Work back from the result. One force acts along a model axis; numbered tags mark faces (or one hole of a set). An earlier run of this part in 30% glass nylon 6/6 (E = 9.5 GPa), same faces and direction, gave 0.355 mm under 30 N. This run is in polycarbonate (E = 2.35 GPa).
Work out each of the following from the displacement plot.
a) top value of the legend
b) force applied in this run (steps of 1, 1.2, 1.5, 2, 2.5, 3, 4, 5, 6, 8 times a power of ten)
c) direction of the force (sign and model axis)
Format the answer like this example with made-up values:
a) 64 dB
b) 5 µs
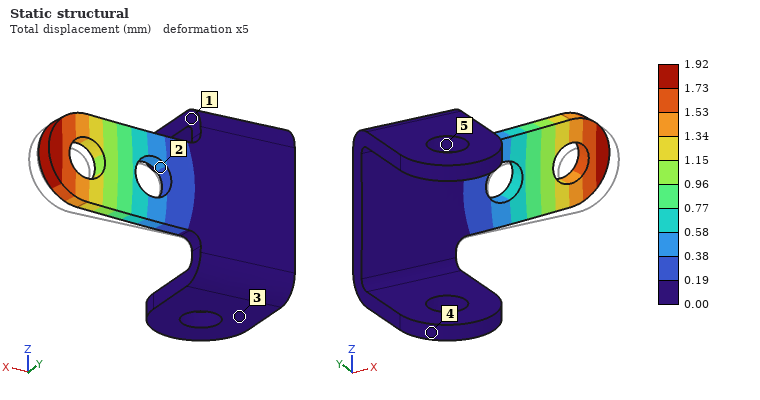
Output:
a) 1.92 mm
b) 40 N
c) +Y
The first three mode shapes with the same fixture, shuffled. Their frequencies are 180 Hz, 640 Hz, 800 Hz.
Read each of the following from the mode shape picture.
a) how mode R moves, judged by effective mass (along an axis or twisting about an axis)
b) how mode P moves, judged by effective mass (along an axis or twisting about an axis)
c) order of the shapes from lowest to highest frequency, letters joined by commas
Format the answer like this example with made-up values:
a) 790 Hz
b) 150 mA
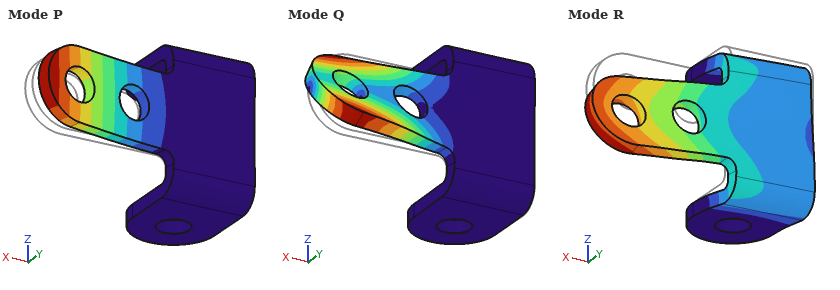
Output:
a) along Z
b) along Y
c) P, R, Q
